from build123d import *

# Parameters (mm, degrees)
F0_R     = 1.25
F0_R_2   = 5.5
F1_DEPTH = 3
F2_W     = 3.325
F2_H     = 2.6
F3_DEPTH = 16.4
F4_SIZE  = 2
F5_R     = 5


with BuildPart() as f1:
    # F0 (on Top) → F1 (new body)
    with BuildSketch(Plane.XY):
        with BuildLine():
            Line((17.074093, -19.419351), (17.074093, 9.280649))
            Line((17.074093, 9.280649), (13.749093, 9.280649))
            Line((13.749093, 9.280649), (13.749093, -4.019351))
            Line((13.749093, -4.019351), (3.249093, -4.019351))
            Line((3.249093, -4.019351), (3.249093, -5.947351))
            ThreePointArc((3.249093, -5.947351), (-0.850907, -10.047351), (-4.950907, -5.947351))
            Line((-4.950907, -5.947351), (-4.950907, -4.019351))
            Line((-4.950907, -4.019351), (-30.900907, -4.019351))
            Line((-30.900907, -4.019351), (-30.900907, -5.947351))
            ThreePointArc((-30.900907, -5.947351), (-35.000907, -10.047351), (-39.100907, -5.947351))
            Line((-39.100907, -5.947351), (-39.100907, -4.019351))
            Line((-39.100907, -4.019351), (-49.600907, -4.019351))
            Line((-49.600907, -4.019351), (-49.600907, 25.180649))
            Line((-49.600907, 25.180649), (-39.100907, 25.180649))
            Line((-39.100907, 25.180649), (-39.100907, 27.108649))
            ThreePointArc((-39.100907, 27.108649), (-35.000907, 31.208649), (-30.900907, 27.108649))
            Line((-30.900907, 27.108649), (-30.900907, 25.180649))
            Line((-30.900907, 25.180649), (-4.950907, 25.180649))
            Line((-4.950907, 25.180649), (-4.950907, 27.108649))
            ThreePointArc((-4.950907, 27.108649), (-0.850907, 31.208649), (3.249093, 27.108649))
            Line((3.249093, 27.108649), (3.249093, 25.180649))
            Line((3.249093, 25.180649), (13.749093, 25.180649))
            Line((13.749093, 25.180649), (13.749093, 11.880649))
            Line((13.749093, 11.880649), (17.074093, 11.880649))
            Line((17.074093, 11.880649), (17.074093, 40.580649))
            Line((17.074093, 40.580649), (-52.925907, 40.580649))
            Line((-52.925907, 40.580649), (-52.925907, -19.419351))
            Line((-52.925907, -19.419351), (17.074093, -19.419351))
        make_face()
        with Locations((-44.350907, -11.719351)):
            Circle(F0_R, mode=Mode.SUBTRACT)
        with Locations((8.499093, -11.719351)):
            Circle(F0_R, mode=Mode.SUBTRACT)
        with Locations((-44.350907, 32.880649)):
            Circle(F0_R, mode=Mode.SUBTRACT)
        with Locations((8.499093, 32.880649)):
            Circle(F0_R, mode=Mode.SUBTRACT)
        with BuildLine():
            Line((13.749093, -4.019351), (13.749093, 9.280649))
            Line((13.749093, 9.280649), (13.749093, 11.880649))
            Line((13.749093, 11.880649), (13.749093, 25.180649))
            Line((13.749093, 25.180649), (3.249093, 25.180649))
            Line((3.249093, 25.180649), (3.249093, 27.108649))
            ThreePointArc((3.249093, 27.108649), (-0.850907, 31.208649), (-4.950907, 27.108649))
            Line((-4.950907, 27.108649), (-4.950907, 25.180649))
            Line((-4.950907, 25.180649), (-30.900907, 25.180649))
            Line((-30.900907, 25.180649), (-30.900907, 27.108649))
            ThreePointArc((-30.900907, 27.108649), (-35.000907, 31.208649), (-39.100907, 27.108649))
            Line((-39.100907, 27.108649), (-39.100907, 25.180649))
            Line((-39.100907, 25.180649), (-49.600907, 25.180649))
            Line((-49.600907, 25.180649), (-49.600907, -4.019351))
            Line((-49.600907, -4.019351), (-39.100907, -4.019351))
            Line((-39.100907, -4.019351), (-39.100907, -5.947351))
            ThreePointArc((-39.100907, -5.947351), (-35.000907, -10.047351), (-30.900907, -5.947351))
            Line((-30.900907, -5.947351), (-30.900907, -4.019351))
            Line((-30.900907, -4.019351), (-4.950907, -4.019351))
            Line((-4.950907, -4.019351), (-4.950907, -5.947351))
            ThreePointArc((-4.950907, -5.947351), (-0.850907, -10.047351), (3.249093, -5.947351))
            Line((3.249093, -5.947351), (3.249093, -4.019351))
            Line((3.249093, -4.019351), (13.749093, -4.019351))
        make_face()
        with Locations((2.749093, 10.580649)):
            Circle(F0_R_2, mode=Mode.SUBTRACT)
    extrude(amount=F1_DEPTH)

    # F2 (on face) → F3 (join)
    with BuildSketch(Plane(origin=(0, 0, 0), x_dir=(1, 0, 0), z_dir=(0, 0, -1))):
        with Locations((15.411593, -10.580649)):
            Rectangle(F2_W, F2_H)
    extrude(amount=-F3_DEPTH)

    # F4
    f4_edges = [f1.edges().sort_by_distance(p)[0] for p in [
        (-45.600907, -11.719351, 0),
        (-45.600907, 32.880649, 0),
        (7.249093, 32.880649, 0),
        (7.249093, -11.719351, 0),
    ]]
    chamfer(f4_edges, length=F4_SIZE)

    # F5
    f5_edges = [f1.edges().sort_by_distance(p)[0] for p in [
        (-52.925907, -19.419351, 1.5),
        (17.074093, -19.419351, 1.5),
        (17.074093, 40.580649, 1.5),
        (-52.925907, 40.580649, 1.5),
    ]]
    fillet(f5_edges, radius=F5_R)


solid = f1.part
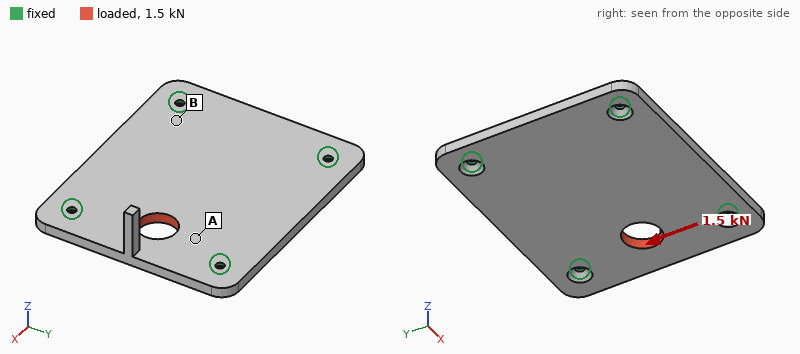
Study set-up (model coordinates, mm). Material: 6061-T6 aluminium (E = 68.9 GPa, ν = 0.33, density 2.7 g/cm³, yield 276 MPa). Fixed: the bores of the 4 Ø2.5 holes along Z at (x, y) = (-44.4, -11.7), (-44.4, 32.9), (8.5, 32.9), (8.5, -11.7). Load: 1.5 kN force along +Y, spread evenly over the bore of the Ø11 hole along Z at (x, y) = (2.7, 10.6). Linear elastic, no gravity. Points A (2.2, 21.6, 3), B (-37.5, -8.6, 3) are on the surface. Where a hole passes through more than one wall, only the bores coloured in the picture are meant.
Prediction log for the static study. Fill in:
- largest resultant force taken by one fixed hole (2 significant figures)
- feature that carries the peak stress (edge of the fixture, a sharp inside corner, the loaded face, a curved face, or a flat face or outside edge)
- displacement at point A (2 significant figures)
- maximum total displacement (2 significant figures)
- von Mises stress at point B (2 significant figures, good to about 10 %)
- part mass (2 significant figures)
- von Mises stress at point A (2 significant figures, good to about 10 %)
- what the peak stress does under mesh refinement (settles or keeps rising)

610 N
edge of the fixture
5.5 µm
11 µm
6.2 MPa
33 g
17 MPa
keeps rising
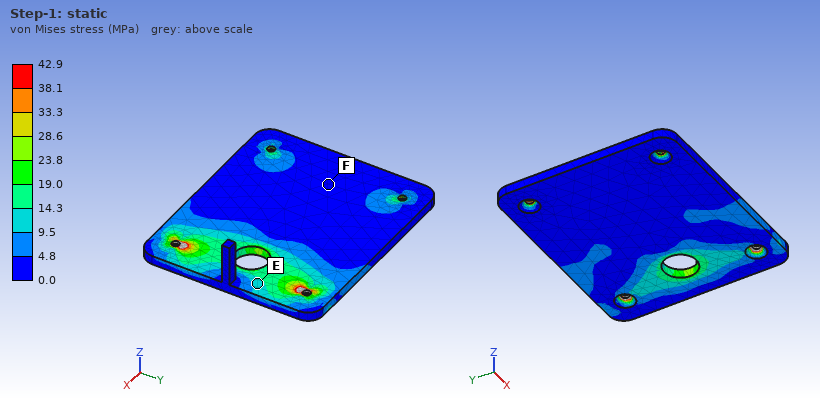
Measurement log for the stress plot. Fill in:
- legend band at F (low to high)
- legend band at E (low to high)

0.0 to 4.8 MPa
9.5 to 14.3 MPa
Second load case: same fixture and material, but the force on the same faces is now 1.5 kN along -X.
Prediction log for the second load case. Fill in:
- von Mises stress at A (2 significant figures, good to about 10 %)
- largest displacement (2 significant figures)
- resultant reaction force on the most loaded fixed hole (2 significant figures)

13 MPa
11 µm
430 N
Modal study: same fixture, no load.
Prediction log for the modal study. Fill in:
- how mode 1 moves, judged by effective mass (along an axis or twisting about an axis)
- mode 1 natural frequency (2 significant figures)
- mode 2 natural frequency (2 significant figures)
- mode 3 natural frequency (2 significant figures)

along Z
3400 Hz
5000 Hz
5100 Hz
